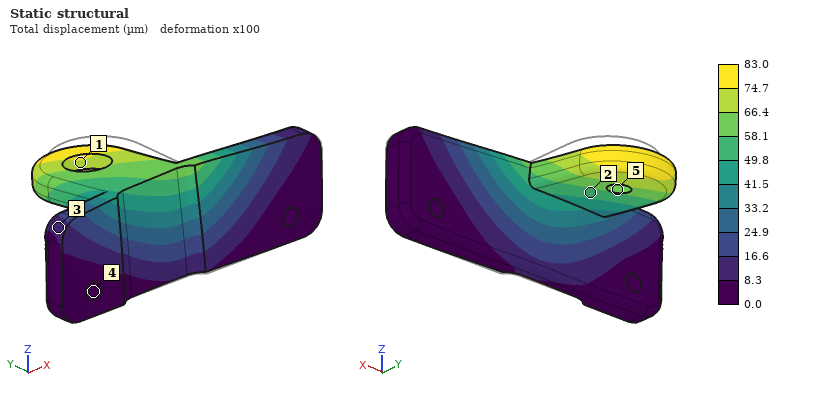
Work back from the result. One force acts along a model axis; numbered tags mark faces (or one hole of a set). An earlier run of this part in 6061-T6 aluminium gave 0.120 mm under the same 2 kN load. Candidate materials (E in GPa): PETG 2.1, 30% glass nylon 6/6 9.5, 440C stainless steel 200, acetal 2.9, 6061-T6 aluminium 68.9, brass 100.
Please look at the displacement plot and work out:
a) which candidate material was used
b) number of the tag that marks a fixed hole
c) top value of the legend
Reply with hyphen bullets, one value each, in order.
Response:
- brass
- 4
- 83.0 µm
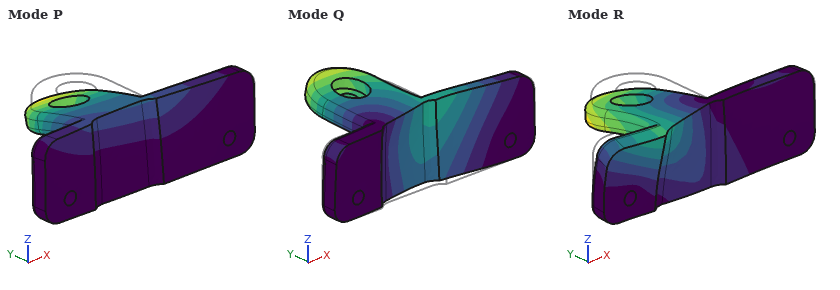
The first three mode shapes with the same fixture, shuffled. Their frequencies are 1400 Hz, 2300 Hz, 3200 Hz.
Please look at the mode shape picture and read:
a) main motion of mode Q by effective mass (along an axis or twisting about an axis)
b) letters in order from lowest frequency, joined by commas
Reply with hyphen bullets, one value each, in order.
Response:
- along Y
- P, Q, R
